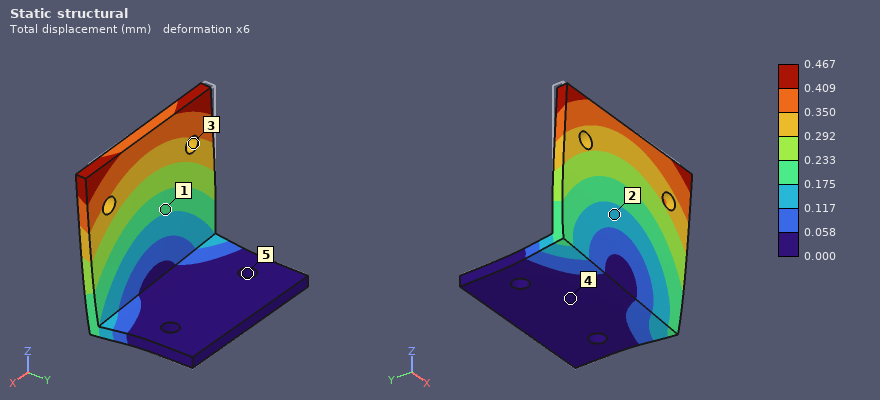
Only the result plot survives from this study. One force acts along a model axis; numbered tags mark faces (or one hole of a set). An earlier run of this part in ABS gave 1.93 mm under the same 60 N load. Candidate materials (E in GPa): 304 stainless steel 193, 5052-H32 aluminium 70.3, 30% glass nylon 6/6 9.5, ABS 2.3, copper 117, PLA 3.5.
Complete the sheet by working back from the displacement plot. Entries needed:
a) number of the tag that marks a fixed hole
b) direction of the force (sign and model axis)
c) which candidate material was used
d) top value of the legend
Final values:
5
+X
30% glass nylon 6/6
0.467 mm
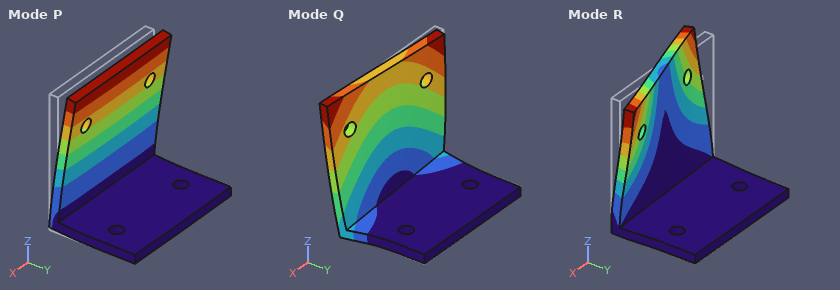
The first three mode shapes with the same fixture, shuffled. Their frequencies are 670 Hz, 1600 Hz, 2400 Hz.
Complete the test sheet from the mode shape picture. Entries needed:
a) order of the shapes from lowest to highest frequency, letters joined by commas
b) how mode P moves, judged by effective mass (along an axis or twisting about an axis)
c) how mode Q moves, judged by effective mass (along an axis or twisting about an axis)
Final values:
P, Q, R
along Y
along X
